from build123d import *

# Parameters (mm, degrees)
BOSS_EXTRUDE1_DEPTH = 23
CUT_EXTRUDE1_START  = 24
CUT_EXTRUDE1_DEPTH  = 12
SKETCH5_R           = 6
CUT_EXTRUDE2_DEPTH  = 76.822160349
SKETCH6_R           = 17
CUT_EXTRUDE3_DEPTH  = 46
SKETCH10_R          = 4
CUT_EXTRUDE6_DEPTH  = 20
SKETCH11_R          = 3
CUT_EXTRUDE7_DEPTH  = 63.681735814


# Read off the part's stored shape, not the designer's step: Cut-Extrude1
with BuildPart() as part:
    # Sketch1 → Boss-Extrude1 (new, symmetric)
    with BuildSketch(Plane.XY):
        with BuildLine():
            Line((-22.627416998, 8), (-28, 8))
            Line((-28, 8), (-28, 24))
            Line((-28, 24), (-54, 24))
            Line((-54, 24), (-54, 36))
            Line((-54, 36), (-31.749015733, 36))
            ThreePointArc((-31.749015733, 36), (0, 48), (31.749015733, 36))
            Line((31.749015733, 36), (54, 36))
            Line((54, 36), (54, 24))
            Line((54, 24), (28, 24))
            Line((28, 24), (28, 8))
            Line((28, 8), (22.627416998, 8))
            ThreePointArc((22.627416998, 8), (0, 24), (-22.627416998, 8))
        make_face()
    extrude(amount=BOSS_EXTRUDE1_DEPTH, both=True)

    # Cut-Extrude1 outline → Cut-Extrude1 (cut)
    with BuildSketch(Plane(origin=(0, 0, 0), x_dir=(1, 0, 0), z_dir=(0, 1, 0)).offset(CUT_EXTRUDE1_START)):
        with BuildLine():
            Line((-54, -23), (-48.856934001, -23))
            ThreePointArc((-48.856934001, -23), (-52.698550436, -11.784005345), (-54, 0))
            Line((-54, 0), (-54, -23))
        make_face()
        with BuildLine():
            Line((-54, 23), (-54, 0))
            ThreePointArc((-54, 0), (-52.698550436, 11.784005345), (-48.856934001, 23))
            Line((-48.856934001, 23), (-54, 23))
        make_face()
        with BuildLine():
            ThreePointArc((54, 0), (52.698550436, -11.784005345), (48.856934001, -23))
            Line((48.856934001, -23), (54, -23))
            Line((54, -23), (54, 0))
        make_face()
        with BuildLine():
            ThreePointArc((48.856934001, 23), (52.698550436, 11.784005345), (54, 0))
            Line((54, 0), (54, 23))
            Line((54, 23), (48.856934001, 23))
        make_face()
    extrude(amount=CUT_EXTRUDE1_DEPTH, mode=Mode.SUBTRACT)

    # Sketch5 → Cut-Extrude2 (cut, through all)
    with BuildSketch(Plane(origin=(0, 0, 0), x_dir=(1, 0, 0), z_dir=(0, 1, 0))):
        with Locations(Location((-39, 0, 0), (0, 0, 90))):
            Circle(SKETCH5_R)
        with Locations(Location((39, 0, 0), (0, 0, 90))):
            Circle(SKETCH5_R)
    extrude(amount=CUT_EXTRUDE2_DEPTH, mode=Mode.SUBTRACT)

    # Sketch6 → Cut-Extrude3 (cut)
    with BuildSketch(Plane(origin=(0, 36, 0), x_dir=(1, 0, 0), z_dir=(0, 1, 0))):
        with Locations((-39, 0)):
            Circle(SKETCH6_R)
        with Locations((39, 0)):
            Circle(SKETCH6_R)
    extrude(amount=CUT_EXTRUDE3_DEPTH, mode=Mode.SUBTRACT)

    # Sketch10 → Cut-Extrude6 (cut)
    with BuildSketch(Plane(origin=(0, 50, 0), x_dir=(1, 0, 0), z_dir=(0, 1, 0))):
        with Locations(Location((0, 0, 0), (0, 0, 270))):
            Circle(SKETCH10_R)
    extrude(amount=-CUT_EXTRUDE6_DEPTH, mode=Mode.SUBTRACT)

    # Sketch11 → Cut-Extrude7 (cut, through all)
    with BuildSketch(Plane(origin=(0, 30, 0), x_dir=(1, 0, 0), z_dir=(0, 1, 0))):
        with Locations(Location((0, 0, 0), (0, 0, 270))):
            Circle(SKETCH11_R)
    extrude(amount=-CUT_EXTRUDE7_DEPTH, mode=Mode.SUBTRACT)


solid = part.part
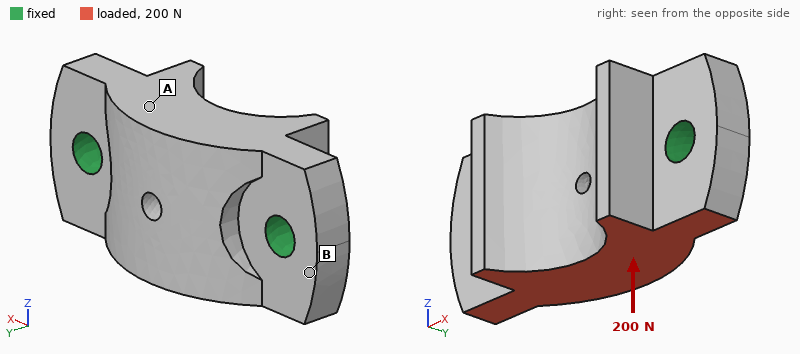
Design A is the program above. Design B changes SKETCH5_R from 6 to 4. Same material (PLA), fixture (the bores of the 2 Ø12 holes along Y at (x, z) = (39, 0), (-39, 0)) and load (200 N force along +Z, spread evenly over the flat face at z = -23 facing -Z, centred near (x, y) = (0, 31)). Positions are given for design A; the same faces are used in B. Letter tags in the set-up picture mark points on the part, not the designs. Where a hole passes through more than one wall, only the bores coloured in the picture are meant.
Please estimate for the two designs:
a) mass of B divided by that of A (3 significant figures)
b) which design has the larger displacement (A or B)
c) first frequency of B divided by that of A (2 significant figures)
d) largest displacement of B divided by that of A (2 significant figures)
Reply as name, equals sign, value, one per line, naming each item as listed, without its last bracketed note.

mass of B divided by that of A = 1.02
which design has the larger displacement = B
first frequency of B divided by that of A = 0.83
largest displacement of B divided by that of A = 1.2
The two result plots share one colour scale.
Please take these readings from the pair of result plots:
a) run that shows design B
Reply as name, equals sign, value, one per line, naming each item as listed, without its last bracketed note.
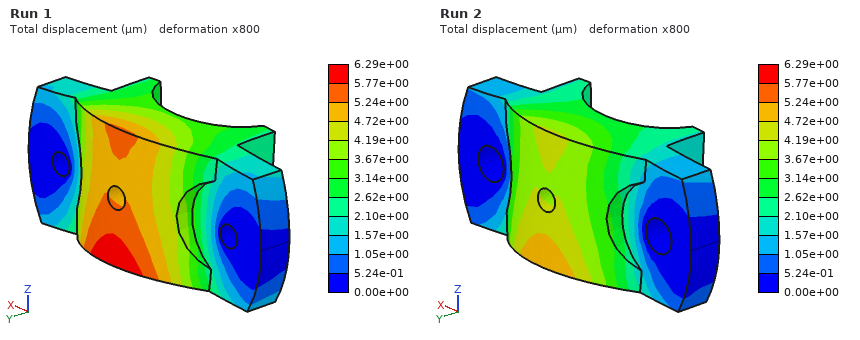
run that shows design B = Run 1
